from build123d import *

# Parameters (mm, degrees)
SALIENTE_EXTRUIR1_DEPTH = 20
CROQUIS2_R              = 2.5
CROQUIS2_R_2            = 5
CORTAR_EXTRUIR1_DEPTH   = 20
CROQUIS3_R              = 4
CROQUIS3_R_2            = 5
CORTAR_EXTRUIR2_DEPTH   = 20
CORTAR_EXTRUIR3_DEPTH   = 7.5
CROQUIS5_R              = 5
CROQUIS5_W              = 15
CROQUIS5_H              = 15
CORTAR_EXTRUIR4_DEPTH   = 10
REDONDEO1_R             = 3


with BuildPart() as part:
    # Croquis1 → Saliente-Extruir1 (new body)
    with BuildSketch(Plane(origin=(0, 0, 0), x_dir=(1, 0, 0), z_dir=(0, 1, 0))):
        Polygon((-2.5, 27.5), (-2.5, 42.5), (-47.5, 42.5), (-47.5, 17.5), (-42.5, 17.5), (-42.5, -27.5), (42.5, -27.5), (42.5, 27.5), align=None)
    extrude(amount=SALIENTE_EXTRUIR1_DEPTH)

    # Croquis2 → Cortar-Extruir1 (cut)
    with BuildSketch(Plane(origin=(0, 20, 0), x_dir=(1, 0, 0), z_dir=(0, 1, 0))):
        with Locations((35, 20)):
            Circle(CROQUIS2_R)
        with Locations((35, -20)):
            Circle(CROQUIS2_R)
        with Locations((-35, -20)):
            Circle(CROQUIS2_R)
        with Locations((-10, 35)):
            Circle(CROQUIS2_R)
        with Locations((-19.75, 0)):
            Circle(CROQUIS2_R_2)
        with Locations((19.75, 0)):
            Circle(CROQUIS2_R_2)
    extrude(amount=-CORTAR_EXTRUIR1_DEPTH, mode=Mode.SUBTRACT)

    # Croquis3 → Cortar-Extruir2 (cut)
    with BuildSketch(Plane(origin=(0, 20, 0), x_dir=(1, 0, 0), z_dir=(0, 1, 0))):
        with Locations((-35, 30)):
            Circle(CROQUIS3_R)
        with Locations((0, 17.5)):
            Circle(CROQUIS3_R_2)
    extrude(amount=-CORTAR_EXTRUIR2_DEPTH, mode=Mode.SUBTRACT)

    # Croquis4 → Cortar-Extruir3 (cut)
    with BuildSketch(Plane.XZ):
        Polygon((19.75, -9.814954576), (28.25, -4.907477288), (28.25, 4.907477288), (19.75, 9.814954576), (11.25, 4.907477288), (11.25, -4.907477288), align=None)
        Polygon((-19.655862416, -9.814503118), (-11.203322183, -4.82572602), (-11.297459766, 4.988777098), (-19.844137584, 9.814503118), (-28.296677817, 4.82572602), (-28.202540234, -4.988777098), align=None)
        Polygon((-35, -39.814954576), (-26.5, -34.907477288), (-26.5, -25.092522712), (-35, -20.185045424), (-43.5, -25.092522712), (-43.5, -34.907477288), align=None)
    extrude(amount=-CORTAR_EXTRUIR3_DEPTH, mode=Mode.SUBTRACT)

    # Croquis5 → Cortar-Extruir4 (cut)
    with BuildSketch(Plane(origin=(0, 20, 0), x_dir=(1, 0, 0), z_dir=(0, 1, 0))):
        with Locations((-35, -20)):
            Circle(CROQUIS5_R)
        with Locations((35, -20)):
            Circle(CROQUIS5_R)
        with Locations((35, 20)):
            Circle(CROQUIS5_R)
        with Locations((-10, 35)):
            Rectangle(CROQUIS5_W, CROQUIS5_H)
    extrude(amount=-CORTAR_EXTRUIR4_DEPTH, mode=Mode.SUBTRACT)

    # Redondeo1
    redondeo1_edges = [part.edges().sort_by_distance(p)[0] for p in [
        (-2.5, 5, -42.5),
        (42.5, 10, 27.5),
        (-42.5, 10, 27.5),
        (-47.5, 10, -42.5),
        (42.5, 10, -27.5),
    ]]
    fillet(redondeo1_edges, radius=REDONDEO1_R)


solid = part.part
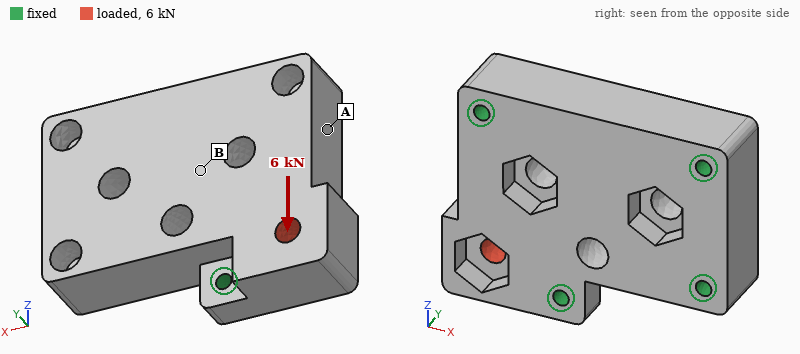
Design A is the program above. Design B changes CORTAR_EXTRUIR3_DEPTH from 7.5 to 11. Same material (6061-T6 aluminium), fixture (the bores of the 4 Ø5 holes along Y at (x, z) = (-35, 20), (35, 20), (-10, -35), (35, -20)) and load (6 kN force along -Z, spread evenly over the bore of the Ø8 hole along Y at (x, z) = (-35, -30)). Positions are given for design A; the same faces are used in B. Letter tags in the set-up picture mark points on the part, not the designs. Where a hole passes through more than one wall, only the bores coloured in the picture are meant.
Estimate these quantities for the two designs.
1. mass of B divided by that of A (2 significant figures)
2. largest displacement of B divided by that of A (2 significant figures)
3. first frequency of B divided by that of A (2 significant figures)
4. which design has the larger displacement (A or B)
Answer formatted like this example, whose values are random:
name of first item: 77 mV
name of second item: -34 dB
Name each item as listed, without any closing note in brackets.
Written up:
mass of B divided by that of A: 0.98
largest displacement of B divided by that of A: 1.2
first frequency of B divided by that of A: 1.0
which design has the larger displacement: B
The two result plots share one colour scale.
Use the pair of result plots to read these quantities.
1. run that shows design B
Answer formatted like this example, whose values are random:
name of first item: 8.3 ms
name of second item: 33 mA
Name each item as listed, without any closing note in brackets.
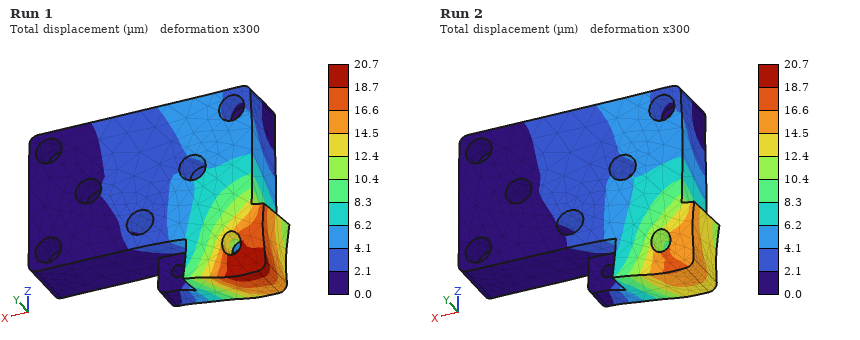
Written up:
run that shows design B: Run 1
